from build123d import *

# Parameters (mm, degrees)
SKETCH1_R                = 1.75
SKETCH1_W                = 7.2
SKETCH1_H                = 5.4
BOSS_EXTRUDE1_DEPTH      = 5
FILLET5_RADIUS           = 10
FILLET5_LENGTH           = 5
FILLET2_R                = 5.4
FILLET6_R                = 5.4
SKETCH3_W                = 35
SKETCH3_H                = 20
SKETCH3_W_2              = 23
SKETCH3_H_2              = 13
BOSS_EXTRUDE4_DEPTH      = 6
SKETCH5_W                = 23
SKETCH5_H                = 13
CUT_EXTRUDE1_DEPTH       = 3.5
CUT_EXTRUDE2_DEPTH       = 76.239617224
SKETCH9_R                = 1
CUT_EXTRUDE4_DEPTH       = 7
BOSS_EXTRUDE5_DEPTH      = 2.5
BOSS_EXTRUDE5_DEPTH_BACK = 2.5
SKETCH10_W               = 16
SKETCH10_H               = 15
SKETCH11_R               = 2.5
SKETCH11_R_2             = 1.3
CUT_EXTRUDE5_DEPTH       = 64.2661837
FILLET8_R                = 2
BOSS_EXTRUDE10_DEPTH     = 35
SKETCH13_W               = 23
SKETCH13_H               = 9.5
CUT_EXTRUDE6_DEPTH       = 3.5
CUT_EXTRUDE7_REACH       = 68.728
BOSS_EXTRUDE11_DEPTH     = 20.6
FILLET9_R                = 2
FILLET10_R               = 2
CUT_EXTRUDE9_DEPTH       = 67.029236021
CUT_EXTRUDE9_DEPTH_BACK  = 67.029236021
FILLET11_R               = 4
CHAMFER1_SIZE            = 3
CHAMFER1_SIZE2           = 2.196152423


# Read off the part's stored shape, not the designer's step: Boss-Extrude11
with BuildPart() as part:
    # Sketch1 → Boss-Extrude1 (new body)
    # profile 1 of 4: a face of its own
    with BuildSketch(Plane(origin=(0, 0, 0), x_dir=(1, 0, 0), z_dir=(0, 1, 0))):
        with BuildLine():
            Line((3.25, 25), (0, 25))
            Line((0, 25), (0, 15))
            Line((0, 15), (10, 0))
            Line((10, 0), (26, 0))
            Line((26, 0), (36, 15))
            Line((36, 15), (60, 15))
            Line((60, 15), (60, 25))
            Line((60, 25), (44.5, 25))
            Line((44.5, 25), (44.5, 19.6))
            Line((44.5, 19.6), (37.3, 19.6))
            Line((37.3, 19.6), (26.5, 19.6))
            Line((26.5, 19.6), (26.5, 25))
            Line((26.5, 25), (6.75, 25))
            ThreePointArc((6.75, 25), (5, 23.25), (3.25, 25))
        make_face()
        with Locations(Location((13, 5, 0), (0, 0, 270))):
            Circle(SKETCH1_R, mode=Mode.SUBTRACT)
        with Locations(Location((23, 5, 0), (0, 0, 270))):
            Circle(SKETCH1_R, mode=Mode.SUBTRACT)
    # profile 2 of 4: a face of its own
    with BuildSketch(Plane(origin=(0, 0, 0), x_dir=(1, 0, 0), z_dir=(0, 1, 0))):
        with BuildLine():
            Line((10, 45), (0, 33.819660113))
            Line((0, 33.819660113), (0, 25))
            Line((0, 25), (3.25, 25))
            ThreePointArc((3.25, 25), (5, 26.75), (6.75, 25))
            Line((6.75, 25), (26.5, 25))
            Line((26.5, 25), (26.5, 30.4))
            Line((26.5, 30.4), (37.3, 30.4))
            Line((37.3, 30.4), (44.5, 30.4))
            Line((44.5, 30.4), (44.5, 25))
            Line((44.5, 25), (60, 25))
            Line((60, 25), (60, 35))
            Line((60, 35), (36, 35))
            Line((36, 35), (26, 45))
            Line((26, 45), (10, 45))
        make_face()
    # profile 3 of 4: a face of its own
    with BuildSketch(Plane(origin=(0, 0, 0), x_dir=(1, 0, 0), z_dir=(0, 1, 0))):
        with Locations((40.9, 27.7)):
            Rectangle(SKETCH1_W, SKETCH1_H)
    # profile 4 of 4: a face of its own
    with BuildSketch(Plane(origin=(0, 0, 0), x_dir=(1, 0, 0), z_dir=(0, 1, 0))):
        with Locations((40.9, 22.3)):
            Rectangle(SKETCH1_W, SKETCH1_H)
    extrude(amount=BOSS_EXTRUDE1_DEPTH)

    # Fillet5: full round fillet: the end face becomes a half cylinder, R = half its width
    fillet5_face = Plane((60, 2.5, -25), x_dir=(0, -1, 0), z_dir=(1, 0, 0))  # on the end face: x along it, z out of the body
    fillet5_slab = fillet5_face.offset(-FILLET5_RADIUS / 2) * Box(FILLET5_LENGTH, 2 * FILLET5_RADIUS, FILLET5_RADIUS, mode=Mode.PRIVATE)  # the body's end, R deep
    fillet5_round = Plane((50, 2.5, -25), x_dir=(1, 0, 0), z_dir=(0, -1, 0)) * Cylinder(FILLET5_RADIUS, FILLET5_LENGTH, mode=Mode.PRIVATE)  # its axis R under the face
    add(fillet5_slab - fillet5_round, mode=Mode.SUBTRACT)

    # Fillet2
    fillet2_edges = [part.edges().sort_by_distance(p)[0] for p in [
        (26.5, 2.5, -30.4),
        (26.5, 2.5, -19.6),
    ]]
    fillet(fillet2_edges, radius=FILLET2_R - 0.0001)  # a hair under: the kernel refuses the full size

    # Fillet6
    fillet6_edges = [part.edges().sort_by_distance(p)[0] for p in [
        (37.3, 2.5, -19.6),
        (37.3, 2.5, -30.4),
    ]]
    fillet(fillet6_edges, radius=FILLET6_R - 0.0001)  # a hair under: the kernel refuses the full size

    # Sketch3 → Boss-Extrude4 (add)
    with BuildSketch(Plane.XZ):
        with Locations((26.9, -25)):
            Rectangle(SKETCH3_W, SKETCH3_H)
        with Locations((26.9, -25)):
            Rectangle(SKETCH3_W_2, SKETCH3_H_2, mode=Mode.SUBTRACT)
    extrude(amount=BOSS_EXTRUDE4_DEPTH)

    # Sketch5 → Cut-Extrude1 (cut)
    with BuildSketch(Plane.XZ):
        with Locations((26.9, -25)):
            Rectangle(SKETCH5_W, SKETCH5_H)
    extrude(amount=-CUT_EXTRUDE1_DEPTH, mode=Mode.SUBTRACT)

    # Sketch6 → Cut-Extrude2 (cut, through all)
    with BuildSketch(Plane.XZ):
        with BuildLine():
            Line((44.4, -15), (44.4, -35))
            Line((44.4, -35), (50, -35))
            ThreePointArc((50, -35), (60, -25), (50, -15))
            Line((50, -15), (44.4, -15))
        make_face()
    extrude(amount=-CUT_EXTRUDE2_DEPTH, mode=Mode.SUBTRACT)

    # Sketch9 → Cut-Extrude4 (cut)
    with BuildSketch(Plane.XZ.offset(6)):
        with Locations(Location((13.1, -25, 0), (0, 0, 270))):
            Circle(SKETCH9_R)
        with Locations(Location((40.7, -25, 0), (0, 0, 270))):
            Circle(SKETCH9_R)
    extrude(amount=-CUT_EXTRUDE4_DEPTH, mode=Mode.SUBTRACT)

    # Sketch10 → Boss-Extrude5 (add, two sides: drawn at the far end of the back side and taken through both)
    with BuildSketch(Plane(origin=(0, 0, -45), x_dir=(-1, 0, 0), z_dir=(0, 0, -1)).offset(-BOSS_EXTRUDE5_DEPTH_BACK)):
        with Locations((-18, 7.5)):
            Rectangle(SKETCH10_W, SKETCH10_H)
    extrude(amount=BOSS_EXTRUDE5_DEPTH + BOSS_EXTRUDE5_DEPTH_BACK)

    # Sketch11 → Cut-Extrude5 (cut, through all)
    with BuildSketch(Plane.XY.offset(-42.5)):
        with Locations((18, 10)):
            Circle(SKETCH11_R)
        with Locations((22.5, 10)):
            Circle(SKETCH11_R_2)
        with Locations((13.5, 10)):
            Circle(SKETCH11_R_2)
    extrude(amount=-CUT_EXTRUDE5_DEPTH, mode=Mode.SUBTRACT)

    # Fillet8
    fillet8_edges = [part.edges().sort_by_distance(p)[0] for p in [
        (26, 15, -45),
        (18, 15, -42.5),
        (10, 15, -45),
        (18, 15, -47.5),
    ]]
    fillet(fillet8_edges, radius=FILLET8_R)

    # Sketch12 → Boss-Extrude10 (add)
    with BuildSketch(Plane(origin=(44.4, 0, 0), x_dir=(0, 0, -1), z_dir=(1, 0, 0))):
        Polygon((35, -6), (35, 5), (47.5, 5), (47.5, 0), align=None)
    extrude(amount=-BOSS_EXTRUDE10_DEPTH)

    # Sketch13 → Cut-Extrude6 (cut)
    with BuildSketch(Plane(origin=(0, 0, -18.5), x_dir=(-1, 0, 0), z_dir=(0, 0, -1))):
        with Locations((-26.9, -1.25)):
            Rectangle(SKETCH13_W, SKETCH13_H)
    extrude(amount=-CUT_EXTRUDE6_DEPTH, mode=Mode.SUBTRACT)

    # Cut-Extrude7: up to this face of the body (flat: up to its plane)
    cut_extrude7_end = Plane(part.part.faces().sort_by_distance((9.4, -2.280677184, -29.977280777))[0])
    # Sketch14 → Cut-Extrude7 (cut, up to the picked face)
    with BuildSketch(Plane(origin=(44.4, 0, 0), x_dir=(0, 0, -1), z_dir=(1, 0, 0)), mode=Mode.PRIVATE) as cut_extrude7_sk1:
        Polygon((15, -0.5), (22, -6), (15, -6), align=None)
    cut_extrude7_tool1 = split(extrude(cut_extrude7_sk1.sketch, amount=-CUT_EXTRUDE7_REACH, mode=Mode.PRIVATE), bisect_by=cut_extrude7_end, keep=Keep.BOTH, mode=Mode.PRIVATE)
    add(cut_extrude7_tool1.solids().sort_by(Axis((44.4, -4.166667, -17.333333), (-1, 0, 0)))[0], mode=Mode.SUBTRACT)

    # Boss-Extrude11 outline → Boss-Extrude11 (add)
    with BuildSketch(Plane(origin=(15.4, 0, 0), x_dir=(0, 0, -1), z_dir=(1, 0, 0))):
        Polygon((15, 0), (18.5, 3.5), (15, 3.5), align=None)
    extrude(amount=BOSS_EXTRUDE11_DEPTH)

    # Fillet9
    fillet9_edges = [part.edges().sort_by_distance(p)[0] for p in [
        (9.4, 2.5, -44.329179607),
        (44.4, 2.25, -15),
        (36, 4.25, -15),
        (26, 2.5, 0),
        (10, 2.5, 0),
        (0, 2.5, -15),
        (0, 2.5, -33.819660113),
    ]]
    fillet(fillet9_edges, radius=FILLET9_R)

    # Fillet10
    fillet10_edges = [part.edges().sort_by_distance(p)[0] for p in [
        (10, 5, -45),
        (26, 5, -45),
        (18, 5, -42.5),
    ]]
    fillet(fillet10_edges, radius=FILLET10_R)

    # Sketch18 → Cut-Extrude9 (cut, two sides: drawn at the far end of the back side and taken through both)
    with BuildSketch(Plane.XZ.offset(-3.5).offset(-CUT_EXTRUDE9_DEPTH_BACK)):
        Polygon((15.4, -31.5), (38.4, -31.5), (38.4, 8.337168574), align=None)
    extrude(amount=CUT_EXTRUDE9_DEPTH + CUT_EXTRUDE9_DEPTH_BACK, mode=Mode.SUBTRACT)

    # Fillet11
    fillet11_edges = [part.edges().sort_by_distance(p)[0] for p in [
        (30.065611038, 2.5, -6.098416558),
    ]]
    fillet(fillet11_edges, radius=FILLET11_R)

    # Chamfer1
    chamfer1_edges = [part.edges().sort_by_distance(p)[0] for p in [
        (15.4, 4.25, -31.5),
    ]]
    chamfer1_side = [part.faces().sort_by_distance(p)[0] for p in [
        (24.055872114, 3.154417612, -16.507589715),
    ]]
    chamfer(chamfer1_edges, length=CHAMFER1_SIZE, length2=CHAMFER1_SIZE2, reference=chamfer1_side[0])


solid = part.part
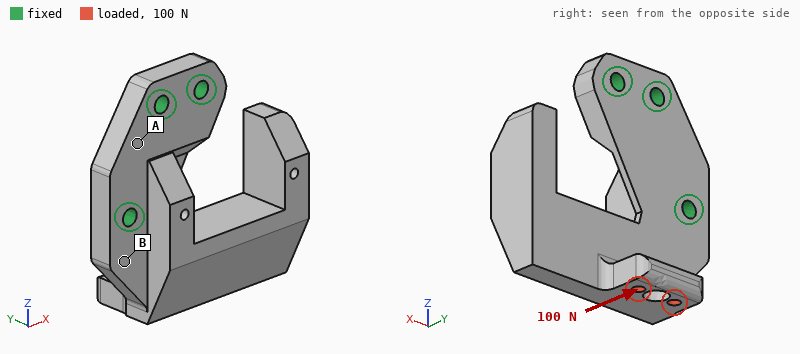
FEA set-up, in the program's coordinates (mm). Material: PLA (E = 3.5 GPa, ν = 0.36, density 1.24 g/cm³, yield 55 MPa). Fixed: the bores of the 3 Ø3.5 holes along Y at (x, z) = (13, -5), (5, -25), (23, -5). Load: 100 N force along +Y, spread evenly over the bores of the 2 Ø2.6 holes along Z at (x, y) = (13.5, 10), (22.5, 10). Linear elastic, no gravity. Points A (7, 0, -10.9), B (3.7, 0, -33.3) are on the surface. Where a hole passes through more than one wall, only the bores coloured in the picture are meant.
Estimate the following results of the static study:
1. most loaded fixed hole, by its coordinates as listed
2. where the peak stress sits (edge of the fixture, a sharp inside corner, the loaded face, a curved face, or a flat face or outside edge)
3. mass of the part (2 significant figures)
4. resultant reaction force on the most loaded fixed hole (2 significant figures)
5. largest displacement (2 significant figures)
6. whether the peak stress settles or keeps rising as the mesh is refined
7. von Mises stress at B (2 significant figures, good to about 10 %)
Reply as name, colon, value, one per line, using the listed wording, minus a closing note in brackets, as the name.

most loaded fixed hole, by its coordinates as listed: (5, -25)
where the peak stress sits: edge of the fixture
mass of the part: 13 g
resultant reaction force on the most loaded fixed hole: 150 N
largest displacement: 0.81 mm
whether the peak stress settles or keeps rising as the mesh is refined: keeps rising
von Mises stress at B: 9.6 MPa
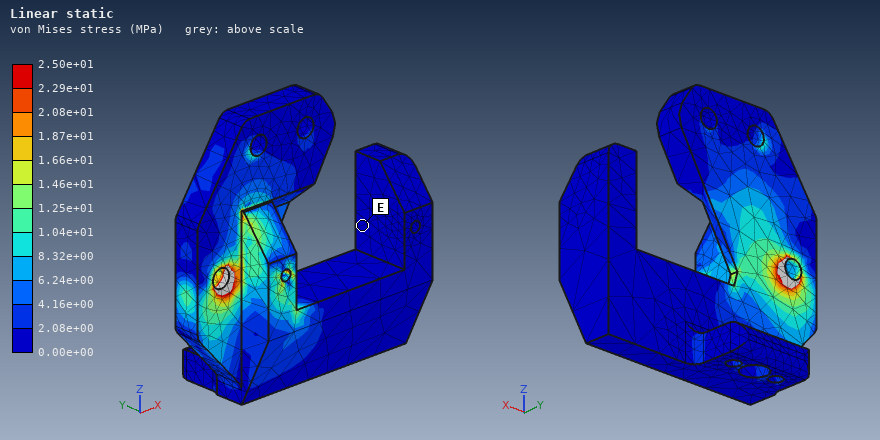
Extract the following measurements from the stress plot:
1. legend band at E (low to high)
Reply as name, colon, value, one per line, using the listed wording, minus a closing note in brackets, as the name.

legend band at E: 0.00e+00 to 2.08e+00 MPa
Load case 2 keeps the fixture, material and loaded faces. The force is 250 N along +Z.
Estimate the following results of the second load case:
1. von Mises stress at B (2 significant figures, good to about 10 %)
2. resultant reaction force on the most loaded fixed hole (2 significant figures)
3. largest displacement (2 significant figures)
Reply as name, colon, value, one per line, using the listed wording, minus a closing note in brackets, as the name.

von Mises stress at B: 13 MPa
resultant reaction force on the most loaded fixed hole: 120 N
largest displacement: 0.69 mm
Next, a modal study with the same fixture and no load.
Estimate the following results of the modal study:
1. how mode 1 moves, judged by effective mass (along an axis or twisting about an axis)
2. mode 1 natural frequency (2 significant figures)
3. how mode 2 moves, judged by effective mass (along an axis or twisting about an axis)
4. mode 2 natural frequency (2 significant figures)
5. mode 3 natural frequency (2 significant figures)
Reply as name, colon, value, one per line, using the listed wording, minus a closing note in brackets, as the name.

how mode 1 moves, judged by effective mass: along Y
mode 1 natural frequency: 630 Hz
how mode 2 moves, judged by effective mass: along Z
mode 2 natural frequency: 1200 Hz
mode 3 natural frequency: 1800 Hz
